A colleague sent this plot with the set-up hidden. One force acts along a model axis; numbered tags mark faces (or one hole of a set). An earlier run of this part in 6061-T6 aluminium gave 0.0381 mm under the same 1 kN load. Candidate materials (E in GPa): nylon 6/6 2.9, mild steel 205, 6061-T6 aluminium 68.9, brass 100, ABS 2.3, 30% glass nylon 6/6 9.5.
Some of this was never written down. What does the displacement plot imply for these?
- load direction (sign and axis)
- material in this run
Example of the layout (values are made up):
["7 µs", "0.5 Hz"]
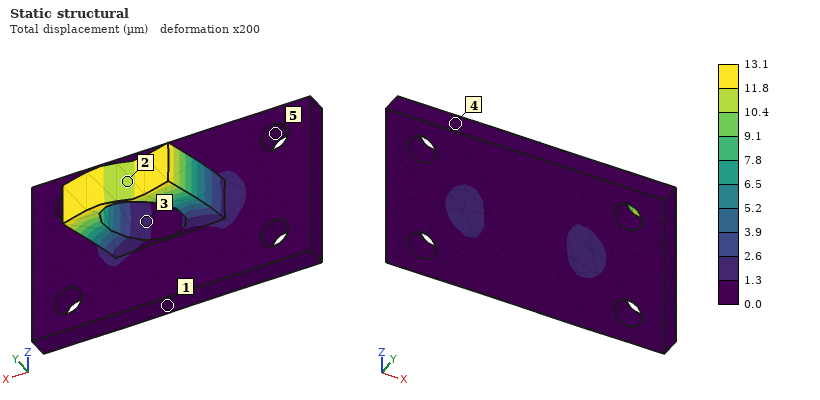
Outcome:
["+X", "mild steel"]
